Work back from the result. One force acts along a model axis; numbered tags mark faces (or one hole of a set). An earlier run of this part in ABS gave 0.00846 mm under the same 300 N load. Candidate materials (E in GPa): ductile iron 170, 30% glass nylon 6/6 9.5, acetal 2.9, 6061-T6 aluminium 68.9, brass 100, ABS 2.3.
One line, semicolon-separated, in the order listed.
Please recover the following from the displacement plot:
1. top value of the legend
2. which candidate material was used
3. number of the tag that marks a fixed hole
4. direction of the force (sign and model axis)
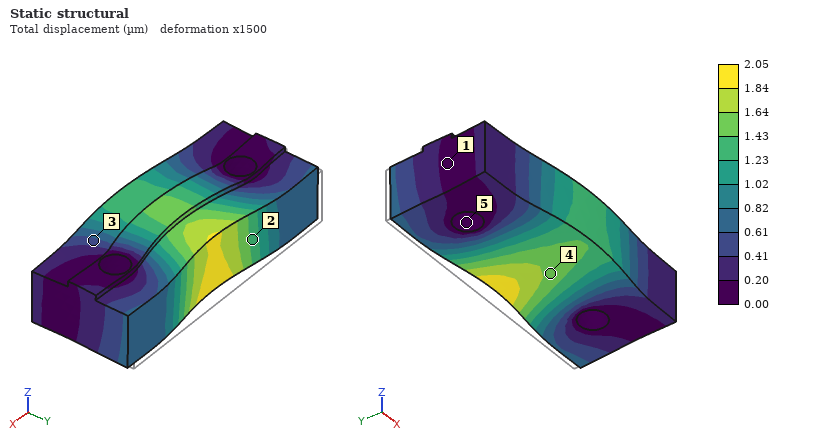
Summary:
2.05 µm; 30% glass nylon 6/6; 5; -Y
